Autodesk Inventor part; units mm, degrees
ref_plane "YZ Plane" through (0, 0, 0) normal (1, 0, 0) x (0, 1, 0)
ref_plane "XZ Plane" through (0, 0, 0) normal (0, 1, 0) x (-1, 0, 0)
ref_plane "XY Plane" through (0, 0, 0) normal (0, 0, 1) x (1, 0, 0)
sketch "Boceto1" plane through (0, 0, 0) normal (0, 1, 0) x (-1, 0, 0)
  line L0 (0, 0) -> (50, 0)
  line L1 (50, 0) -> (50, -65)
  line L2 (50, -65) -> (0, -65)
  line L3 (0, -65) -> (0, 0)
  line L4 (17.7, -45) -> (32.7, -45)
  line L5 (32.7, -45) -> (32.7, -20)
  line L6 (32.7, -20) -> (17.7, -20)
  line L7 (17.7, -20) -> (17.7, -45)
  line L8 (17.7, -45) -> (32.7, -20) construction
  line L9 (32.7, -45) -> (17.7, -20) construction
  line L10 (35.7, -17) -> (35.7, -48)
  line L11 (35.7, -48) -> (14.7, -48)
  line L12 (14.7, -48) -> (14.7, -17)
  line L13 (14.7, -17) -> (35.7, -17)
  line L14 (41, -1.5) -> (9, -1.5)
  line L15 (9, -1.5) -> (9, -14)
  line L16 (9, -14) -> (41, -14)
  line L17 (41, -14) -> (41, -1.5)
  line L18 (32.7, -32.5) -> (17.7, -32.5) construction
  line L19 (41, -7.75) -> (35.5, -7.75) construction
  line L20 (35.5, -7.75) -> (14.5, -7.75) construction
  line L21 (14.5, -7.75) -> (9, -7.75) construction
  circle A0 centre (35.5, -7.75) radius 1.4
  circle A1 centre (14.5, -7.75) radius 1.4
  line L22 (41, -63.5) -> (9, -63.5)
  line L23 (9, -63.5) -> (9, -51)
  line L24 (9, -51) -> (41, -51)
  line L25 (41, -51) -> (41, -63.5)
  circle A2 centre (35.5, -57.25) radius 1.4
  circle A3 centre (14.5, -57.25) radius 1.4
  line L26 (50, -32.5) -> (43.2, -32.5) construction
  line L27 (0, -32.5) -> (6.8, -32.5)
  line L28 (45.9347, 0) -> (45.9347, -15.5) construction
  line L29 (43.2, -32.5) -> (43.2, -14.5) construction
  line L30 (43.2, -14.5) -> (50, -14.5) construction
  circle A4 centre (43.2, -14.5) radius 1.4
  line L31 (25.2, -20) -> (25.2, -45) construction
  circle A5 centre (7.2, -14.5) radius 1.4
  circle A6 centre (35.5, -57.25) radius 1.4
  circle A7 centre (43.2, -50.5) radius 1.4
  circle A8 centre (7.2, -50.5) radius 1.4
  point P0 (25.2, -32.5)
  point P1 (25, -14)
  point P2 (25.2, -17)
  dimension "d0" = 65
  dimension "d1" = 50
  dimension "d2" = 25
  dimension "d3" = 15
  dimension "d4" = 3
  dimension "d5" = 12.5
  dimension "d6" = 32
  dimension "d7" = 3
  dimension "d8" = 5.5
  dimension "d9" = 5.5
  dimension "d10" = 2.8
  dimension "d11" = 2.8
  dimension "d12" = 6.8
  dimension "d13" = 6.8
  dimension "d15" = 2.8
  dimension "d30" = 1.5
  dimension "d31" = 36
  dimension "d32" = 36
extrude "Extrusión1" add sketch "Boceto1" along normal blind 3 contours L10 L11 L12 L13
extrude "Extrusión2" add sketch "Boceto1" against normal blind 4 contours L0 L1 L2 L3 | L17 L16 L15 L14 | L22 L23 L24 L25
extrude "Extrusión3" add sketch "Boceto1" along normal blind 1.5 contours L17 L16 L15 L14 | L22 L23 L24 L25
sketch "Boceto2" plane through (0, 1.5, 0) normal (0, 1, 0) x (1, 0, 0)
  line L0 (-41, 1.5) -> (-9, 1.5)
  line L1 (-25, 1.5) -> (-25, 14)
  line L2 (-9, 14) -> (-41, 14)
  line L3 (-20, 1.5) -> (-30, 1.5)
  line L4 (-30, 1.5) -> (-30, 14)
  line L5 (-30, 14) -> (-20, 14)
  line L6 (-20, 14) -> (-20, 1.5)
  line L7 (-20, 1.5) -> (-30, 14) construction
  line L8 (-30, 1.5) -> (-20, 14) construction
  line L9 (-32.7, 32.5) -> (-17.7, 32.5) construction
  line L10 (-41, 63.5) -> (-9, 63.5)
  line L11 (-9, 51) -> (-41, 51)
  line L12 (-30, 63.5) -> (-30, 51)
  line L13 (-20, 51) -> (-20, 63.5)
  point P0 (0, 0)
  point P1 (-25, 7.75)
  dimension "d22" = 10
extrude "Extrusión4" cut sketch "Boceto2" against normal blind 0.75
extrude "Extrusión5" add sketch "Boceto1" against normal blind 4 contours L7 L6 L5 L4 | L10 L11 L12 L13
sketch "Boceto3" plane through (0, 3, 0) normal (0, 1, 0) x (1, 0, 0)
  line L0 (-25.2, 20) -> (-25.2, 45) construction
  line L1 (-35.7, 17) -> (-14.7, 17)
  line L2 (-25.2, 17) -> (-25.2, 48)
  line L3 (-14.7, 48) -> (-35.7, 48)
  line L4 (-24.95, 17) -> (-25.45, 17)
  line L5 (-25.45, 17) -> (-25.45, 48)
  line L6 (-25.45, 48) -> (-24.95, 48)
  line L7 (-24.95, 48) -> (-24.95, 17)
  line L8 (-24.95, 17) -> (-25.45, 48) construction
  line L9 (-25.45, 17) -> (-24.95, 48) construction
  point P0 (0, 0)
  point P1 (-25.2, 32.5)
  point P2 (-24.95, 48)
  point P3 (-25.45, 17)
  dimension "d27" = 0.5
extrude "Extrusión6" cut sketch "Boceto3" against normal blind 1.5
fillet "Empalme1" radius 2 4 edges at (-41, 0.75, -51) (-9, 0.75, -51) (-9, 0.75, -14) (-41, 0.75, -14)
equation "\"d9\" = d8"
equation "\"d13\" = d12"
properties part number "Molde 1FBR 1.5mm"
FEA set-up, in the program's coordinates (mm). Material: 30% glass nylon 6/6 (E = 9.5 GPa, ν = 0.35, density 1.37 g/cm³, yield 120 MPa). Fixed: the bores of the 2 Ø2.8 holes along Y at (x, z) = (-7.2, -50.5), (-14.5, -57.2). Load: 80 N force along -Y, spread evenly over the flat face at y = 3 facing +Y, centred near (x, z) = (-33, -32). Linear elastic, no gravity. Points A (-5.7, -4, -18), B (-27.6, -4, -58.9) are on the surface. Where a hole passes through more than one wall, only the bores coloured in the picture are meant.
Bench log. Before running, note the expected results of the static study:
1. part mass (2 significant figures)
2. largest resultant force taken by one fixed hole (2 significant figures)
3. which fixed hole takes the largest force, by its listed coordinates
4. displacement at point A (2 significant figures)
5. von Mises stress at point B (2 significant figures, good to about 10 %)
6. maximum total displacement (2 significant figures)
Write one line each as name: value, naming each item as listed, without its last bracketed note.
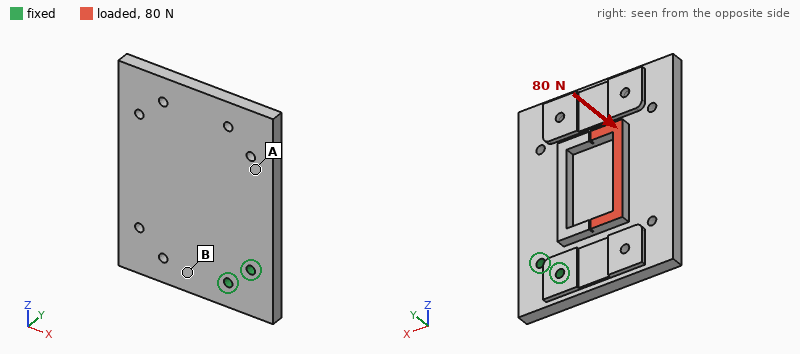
part mass: 20 g
largest resultant force taken by one fixed hole: 65 N
which fixed hole takes the largest force, by its listed coordinates: (-14.5, -57.2)
displacement at point A: 0.21 mm
von Mises stress at point B: 10 MPa
maximum total displacement: 0.82 mm
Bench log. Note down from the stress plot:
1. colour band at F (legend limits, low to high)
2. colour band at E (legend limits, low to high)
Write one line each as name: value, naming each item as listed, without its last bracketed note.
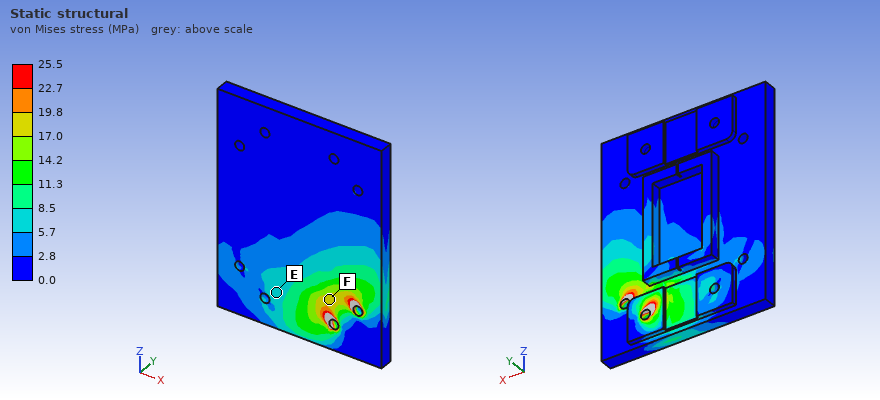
colour band at F: 17.0 to 19.8 MPa
colour band at E: 5.7 to 8.5 MPa
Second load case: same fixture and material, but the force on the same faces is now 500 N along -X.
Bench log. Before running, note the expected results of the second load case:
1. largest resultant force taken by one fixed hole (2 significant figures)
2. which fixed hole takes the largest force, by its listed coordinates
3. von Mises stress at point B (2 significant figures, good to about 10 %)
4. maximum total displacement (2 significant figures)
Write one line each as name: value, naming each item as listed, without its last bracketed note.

largest resultant force taken by one fixed hole: 1.0 kN
which fixed hole takes the largest force, by its listed coordinates: (-7.2, -50.5)
von Mises stress at point B: 16 MPa
maximum total displacement: 0.82 mm
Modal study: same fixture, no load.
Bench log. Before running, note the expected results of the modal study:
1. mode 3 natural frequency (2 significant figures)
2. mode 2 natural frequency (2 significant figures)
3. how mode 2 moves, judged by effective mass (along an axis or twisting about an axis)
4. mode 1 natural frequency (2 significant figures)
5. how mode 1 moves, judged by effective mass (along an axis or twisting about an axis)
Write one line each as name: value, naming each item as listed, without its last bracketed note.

mode 3 natural frequency: 1700 Hz
mode 2 natural frequency: 1200 Hz
how mode 2 moves, judged by effective mass: twisting about Z
mode 1 natural frequency: 510 Hz
how mode 1 moves, judged by effective mass: along Y
